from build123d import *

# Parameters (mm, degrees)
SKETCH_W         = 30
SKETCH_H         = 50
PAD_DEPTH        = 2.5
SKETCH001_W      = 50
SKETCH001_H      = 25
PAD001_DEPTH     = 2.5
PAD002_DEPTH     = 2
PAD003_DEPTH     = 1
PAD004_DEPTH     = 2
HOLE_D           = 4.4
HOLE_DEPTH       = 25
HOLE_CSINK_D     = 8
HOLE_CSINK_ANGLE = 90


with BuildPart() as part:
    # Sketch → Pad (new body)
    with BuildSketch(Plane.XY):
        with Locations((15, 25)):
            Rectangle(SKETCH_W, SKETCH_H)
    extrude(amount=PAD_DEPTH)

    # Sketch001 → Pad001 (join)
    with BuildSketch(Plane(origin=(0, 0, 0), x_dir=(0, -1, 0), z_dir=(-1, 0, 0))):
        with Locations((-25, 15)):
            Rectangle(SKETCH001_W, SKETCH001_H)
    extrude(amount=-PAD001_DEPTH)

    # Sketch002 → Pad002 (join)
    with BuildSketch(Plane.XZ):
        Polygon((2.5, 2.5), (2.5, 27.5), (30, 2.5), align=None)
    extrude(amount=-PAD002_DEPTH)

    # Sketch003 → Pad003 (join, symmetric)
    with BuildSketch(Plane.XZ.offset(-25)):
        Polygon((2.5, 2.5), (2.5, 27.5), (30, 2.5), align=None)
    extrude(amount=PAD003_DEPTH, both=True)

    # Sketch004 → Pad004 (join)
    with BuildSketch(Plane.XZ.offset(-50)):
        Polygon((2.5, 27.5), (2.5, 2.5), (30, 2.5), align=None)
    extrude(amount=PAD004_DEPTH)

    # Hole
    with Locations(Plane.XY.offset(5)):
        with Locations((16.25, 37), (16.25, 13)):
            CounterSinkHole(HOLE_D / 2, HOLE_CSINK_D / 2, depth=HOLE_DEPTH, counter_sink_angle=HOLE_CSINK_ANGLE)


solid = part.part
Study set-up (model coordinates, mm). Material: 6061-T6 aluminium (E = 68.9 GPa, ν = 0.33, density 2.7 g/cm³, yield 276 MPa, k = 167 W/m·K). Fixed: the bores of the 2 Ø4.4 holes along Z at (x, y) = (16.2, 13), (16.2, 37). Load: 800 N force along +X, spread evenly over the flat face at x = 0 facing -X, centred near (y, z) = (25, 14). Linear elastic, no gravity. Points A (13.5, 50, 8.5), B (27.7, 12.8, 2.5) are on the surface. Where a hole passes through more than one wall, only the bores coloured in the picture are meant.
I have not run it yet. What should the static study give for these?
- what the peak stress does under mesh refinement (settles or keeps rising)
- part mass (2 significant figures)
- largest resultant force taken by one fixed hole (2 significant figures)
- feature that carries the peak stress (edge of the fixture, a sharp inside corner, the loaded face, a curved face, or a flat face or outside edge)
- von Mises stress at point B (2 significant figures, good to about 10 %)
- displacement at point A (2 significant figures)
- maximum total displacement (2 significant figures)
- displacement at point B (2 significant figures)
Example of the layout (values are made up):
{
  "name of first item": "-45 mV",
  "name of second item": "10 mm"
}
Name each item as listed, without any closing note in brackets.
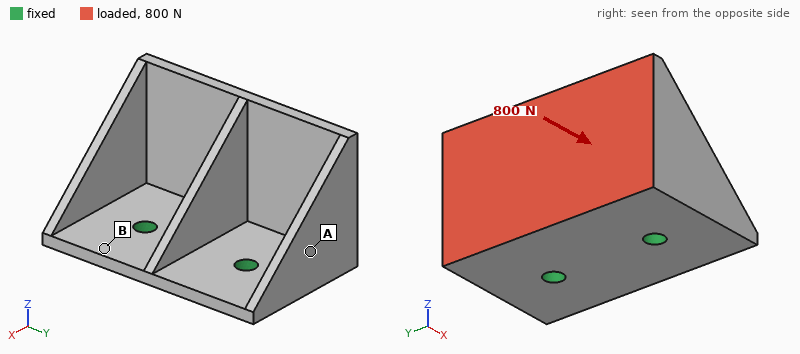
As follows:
{
  "what the peak stress does under mesh refinement": "keeps rising",
  "part mass": "24 g",
  "largest resultant force taken by one fixed hole": "400 N",
  "feature that carries the peak stress": "edge of the fixture",
  "von Mises stress at point B": "40 MPa",
  "displacement at point A": "0.048 mm",
  "maximum total displacement": "0.21 mm",
  "displacement at point B": "0.047 mm"
}
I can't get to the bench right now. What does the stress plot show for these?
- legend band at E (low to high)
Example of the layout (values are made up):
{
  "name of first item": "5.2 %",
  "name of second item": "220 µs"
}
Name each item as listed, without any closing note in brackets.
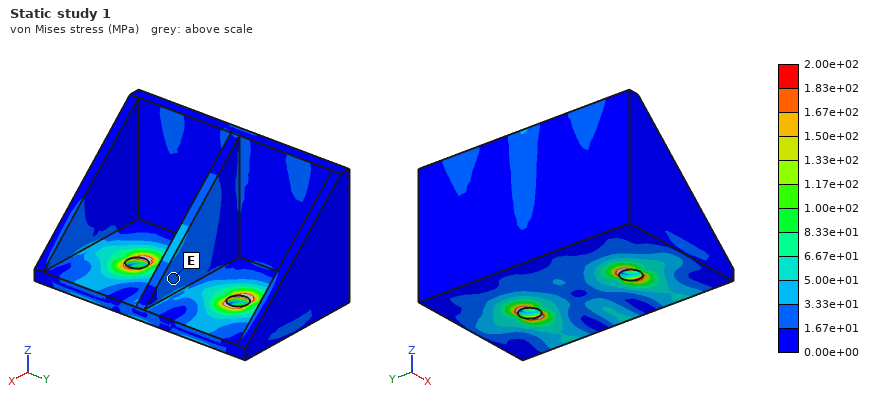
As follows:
{
  "legend band at E": "1.67e+01 to 3.33e+01 MPa"
}
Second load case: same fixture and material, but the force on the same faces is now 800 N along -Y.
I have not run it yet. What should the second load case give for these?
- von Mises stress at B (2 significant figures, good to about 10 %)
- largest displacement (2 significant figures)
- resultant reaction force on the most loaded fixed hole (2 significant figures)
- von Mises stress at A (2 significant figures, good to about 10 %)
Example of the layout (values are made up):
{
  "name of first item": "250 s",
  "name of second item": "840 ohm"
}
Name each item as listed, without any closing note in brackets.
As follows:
{
  "von Mises stress at B": "14 MPa",
  "largest displacement": "0.17 mm",
  "resultant reaction force on the most loaded fixed hole": "700 N",
  "von Mises stress at A": "14 MPa"
}
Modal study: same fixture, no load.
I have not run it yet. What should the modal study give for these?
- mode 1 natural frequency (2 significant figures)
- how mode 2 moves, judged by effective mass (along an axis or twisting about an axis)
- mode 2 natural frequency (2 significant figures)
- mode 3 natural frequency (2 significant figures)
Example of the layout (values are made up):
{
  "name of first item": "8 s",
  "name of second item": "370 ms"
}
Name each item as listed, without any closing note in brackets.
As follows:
{
  "mode 1 natural frequency": "2700 Hz",
  "how mode 2 moves, judged by effective mass": "along Y",
  "mode 2 natural frequency": "2900 Hz",
  "mode 3 natural frequency": "6300 Hz"
}
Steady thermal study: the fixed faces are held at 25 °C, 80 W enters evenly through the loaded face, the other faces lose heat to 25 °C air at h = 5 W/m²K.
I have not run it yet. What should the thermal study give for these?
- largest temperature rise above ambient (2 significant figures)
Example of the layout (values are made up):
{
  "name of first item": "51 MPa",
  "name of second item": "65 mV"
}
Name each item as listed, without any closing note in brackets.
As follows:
{
  "largest temperature rise above ambient": "74 K"
}
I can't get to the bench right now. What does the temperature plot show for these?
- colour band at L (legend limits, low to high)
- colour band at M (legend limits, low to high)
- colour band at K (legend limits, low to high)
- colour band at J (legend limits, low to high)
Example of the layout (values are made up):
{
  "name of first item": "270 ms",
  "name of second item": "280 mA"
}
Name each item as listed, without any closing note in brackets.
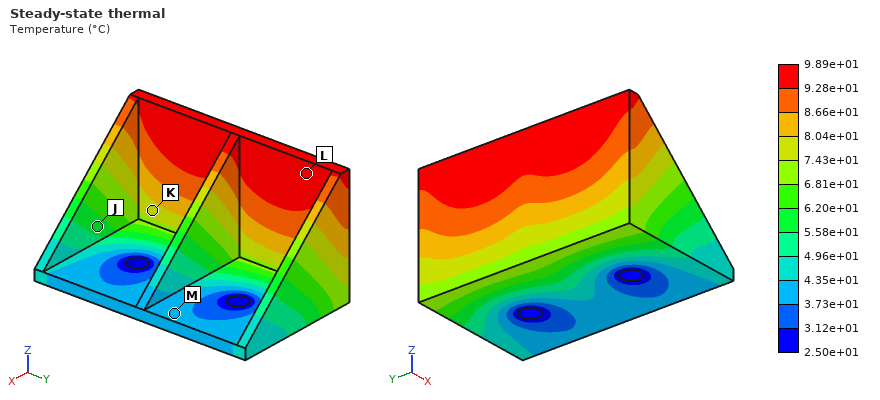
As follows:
{
  "colour band at L": "9.28e+01 to 9.89e+01 °C",
  "colour band at M": "3.73e+01 to 4.35e+01 °C",
  "colour band at K": "7.43e+01 to 8.04e+01 °C",
  "colour band at J": "5.58e+01 to 6.20e+01 °C"
}
